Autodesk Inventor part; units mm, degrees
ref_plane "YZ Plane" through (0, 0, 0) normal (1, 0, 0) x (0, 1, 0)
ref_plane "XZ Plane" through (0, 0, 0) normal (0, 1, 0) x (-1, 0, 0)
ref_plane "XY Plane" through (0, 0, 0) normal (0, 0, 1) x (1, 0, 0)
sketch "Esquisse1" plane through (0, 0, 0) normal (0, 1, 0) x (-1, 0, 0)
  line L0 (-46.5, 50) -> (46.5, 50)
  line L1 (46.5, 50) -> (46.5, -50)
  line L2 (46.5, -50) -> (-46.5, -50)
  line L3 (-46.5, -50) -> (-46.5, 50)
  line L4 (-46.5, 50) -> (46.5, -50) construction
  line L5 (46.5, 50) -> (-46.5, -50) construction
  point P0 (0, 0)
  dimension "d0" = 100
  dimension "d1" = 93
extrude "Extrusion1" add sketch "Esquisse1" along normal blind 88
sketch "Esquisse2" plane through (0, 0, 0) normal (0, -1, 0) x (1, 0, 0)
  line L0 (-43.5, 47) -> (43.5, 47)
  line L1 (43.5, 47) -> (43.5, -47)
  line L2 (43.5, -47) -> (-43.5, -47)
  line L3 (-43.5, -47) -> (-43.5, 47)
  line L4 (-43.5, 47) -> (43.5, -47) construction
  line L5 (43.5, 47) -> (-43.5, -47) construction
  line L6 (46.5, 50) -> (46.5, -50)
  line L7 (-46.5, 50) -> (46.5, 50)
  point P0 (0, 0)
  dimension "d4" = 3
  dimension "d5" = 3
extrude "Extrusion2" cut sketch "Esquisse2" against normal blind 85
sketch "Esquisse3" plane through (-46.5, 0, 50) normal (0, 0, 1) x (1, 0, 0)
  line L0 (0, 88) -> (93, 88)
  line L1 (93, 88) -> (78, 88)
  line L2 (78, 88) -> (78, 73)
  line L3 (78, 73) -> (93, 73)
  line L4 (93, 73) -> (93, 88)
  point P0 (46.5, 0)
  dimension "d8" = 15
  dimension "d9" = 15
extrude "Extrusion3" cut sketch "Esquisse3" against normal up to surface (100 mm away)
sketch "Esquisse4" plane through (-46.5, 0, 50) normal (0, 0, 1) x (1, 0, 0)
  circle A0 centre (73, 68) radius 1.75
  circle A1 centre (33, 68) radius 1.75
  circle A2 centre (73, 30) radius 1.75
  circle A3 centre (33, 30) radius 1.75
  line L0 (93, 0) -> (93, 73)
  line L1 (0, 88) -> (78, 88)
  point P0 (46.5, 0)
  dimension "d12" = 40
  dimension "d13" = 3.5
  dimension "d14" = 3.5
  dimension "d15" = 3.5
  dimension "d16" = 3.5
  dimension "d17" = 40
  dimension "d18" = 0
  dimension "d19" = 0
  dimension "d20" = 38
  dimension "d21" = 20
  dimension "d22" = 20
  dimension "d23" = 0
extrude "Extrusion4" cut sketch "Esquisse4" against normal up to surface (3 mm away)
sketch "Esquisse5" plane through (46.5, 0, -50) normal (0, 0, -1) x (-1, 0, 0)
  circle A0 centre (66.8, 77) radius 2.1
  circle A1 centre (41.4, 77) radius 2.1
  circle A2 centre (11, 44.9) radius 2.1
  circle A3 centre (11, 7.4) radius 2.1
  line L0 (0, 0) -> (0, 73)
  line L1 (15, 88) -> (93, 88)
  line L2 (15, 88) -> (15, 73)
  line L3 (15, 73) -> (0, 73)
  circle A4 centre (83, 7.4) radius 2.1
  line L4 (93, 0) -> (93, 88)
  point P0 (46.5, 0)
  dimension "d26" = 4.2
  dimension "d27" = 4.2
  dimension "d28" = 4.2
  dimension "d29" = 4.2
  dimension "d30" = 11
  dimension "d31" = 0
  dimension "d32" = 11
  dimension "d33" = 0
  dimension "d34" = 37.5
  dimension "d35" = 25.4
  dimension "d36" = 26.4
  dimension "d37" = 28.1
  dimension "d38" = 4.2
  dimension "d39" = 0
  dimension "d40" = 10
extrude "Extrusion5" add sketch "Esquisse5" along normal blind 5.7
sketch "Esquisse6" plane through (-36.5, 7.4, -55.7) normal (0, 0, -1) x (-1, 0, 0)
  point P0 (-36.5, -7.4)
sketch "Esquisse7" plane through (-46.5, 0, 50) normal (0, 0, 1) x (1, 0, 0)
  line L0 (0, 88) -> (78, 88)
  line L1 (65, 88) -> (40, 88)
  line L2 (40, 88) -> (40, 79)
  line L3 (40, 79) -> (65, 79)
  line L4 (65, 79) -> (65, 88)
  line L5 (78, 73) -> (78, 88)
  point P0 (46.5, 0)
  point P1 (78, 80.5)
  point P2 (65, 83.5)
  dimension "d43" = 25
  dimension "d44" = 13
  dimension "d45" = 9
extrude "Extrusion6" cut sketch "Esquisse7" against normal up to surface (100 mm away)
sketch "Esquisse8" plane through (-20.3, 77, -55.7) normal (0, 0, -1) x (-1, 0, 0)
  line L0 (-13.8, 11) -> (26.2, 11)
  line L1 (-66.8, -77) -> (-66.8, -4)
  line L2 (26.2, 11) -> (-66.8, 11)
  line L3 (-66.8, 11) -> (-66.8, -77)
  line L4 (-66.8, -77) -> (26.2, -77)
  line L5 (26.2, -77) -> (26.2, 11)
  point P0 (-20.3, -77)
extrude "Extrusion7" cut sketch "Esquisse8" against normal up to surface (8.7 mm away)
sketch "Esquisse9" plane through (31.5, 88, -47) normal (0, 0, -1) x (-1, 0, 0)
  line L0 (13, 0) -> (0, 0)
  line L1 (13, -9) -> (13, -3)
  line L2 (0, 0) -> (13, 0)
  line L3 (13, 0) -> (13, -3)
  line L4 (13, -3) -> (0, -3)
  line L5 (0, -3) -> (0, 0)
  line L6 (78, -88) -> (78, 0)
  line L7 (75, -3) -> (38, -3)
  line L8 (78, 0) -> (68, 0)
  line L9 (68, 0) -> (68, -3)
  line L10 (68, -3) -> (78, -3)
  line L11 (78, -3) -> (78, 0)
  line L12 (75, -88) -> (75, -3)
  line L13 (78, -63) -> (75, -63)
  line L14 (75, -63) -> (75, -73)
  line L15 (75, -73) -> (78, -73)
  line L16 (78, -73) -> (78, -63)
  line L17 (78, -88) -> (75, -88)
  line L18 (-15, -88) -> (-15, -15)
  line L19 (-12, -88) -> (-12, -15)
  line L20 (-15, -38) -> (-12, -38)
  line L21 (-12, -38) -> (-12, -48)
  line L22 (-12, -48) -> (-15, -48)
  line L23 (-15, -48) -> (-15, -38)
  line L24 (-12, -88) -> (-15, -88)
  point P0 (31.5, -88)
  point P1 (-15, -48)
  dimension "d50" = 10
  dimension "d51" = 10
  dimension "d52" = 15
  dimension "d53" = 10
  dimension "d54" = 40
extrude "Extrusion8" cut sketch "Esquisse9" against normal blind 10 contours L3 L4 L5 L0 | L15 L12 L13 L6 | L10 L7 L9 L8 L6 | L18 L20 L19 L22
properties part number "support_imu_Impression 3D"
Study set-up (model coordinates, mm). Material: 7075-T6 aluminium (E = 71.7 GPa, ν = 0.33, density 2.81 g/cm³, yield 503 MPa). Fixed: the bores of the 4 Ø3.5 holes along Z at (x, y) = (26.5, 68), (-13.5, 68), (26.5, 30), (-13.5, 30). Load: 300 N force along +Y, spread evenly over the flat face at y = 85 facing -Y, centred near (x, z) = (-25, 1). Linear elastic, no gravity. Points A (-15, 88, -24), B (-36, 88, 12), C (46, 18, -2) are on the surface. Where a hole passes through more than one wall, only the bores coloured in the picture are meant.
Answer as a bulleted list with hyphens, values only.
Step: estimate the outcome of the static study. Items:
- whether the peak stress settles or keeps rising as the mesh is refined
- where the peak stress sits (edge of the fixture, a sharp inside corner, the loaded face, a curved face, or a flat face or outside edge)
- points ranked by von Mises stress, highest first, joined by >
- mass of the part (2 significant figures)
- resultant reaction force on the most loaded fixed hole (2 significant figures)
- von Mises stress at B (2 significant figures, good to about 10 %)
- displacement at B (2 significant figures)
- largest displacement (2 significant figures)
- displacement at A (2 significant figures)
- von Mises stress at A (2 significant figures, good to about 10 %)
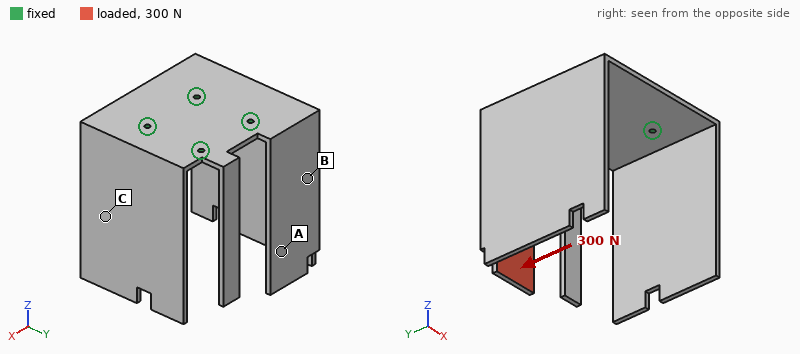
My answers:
- keeps rising
- edge of the fixture
- B > A > C
- 230 g
- 370 N
- 28 MPa
- 0.49 mm
- 1.5 mm
- 1.1 mm
- 16 MPa
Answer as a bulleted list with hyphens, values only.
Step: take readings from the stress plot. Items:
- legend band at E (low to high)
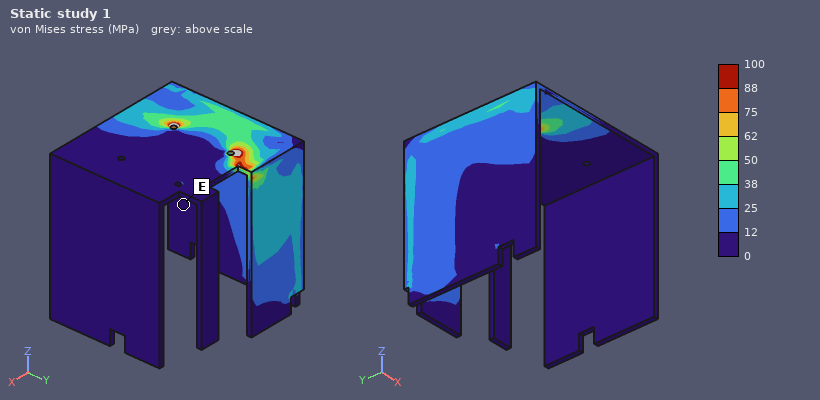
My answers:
- 0 to 12 MPa
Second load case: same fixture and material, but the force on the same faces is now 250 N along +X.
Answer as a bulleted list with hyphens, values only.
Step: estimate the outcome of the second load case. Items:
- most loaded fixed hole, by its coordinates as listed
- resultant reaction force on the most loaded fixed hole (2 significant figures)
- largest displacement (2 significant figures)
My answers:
- (-13.5, 68)
- 240 N
- 1.8 mm
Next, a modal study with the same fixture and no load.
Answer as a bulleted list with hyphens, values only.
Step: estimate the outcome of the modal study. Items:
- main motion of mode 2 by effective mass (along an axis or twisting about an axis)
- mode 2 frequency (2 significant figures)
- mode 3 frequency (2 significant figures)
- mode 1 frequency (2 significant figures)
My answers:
- along X
- 230 Hz
- 260 Hz
- 210 Hz
